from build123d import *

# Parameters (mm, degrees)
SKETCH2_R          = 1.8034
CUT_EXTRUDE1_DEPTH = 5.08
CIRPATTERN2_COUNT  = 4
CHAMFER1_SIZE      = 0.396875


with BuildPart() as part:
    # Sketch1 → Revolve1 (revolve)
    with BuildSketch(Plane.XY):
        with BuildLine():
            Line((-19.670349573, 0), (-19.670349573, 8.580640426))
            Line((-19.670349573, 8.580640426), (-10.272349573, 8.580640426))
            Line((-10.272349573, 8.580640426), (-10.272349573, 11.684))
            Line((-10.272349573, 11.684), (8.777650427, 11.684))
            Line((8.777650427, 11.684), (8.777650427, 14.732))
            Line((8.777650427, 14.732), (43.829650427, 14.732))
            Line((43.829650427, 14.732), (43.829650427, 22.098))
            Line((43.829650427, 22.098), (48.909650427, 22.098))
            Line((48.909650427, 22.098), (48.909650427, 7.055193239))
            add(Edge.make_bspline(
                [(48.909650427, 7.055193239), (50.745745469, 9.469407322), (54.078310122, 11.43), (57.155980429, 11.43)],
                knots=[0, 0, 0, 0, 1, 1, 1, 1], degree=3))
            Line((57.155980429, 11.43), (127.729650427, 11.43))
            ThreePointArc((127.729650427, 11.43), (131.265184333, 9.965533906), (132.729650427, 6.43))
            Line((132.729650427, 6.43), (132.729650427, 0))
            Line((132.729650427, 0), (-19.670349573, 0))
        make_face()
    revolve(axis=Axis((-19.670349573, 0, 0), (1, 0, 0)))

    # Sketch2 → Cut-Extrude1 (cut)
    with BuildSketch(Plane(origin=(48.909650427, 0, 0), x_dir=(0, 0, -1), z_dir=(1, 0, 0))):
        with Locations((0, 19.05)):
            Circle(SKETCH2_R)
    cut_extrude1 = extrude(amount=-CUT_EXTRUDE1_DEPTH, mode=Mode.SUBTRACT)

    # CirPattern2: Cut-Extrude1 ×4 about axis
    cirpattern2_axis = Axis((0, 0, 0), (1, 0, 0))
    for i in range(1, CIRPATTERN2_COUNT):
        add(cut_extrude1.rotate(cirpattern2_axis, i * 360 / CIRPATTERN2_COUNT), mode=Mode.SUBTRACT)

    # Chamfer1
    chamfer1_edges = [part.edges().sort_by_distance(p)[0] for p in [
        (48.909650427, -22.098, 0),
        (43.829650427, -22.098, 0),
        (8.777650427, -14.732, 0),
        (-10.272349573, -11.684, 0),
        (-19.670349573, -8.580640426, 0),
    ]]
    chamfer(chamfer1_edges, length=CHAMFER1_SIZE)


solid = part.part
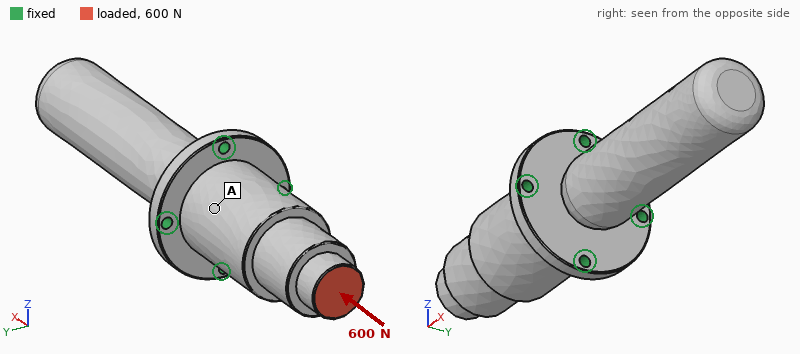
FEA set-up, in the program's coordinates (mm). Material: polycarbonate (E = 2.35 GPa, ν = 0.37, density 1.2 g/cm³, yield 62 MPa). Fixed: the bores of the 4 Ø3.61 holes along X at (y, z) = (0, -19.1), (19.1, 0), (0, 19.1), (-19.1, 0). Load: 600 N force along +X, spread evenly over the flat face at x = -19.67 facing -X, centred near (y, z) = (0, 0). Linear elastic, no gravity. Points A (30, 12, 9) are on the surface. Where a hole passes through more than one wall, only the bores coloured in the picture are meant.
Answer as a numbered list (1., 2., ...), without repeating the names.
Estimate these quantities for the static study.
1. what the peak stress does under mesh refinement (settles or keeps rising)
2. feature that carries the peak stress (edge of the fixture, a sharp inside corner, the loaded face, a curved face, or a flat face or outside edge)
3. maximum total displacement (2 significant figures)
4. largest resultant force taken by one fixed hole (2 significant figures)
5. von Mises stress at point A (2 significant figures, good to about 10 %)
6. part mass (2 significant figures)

1. keeps rising
2. edge of the fixture
3. 65 µm
4. 160 N
5. 0.84 MPa
6. 90 g
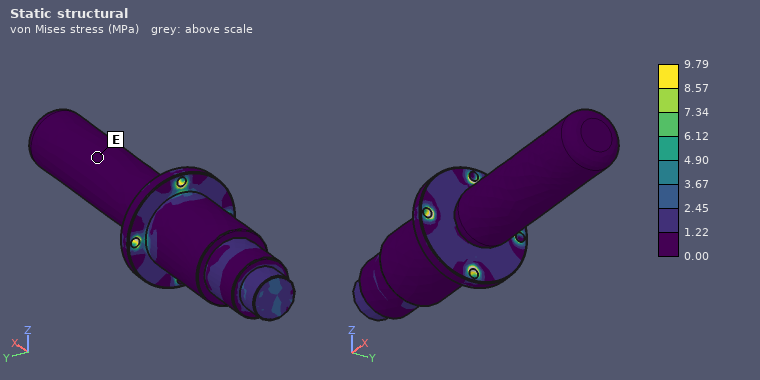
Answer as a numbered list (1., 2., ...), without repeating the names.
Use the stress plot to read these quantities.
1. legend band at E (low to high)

1. 0.00 to 1.22 MPa
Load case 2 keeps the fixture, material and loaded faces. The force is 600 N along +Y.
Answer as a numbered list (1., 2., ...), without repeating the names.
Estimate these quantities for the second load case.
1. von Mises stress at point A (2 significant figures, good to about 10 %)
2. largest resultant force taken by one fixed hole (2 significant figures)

1. 9.3 MPa
2. 1.1 kN
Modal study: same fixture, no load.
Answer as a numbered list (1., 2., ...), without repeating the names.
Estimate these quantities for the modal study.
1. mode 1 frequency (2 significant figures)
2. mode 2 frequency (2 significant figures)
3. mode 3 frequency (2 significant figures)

1. 350 Hz
2. 350 Hz
3. 1100 Hz
